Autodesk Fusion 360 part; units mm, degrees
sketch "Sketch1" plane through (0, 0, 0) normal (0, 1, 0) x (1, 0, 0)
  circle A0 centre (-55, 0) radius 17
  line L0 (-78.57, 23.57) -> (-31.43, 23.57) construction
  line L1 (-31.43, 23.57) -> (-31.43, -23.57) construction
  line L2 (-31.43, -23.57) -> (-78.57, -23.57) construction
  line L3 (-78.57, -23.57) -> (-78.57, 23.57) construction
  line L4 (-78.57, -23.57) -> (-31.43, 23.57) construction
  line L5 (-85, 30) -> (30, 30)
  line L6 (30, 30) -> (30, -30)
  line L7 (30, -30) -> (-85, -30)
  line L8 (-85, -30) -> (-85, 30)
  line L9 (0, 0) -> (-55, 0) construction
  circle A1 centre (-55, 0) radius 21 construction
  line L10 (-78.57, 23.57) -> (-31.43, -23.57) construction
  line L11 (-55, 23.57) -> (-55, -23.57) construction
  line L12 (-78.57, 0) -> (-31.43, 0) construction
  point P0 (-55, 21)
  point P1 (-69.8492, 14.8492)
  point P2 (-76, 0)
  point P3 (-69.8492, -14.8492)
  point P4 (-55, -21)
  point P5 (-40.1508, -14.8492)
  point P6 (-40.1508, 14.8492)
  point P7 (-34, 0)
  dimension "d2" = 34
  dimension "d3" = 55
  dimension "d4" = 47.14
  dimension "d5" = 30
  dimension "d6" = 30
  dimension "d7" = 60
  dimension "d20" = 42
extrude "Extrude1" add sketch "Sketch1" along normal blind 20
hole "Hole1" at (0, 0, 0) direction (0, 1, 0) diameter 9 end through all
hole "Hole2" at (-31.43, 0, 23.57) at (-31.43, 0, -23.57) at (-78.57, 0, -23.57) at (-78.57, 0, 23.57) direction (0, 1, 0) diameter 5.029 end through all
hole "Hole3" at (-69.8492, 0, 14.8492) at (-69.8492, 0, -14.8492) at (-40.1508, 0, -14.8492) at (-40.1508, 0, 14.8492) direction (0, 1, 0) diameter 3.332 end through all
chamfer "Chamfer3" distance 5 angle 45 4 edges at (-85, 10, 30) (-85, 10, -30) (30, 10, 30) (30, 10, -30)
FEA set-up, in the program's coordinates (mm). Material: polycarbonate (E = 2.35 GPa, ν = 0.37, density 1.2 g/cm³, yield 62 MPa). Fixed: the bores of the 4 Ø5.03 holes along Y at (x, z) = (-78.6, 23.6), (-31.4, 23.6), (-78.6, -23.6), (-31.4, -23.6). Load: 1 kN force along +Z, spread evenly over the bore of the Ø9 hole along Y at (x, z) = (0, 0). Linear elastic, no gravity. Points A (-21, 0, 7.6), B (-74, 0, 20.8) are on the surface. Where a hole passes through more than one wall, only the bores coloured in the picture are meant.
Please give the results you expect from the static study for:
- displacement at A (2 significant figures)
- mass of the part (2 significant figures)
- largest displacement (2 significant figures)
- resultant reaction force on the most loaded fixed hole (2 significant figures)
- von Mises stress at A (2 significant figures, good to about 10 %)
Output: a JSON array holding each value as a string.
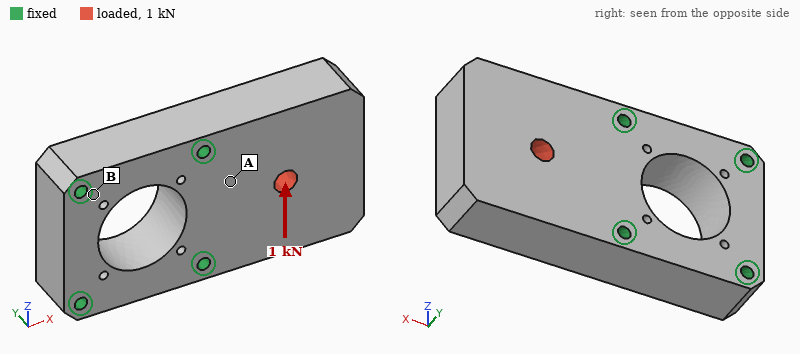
["15 µm", "140 g", "72 µm", "790 N", "1.7 MPa"]
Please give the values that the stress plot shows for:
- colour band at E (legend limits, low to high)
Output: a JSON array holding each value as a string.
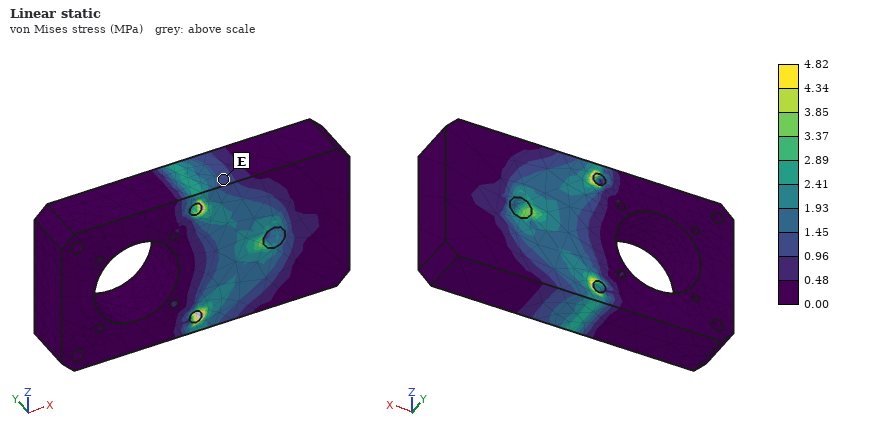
["0.96 to 1.45 MPa"]
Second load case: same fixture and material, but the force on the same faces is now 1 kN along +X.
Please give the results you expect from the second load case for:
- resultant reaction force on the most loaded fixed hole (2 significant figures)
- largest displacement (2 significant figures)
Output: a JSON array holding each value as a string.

["490 N", "26 µm"]
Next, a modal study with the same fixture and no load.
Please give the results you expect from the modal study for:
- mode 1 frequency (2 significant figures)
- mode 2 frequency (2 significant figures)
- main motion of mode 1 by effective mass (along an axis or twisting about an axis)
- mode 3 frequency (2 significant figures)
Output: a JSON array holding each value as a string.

["960 Hz", "2200 Hz", "along Y", "2300 Hz"]
